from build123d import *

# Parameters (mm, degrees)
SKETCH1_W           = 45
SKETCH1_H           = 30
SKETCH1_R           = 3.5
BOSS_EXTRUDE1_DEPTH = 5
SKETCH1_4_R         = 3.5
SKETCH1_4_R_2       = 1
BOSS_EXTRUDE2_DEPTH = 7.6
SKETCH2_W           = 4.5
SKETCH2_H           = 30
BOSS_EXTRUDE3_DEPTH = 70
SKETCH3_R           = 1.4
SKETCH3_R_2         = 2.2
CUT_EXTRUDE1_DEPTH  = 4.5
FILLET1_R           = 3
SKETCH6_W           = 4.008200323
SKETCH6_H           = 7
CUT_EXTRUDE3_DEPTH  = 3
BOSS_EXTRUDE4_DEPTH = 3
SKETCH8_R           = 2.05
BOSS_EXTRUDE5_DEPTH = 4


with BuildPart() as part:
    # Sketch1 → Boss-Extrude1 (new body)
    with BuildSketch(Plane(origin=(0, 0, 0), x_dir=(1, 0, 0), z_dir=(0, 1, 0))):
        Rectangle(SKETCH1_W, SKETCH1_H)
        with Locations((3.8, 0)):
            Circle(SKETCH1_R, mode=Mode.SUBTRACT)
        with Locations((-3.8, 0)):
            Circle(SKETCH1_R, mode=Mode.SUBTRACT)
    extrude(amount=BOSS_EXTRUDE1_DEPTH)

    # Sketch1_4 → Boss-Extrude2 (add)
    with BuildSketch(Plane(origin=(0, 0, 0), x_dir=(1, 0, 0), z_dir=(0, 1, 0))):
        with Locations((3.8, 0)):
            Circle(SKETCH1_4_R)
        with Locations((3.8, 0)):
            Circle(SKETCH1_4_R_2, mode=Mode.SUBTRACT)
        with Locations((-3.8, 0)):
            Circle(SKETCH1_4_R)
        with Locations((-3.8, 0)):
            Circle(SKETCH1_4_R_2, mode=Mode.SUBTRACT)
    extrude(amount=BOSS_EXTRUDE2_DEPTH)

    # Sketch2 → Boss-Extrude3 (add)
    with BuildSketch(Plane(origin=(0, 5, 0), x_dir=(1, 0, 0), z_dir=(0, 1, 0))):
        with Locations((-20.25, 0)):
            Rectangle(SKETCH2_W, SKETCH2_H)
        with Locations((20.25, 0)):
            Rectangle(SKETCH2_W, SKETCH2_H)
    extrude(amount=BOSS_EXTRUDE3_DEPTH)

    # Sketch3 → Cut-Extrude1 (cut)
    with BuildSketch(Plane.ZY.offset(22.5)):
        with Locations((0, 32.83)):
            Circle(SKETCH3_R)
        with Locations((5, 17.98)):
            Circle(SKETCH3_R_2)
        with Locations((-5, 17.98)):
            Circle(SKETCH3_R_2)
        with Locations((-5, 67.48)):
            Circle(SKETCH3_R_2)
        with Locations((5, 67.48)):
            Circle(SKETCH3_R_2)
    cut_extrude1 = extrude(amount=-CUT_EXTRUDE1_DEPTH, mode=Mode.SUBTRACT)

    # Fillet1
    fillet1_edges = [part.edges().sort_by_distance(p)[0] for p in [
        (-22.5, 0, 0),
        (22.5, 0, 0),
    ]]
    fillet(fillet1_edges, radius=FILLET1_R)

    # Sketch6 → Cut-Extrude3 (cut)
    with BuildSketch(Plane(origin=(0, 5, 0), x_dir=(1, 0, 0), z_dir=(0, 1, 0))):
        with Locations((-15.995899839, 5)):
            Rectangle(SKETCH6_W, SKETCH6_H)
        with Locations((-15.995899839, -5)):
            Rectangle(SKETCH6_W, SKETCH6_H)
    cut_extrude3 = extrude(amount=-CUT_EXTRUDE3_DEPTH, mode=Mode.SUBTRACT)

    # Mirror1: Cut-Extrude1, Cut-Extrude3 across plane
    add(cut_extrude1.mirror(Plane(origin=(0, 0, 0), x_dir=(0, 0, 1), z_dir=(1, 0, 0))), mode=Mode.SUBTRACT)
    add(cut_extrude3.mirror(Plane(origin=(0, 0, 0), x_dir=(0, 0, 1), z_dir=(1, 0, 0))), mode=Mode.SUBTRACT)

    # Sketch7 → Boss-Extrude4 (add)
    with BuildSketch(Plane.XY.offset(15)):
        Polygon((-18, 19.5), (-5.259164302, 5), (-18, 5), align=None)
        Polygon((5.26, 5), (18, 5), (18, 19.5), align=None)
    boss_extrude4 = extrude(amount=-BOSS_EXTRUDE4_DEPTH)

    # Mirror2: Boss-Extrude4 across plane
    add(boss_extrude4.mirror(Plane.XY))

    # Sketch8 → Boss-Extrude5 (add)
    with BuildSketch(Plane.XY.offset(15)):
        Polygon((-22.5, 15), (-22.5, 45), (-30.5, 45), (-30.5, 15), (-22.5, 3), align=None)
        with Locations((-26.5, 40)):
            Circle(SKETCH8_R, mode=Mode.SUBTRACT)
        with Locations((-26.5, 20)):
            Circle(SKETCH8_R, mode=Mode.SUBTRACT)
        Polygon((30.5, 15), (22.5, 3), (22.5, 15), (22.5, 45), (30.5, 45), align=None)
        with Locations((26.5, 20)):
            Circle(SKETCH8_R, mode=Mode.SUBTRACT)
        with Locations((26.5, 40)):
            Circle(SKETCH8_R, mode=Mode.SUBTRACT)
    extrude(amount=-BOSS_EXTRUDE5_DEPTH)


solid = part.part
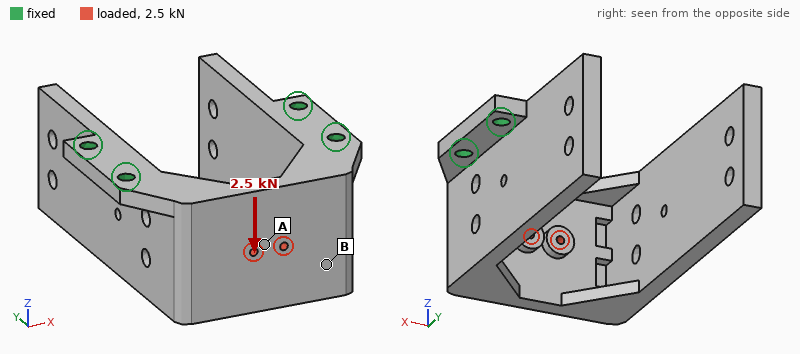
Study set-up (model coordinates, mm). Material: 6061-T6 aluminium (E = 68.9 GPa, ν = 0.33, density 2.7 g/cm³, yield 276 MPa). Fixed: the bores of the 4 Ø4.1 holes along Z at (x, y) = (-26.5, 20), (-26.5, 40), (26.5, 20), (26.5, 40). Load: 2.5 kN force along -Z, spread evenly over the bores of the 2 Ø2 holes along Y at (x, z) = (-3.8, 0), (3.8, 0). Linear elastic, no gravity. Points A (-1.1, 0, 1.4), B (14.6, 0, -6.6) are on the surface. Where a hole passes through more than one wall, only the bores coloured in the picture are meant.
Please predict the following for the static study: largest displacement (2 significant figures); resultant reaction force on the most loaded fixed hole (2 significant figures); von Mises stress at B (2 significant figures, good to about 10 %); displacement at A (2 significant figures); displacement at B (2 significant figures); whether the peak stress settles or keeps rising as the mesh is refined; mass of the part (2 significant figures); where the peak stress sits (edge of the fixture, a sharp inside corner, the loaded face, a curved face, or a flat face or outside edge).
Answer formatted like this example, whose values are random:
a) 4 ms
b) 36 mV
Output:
a) 82 µm
b) 2.1 kN
c) 28 MPa
d) 72 µm
e) 69 µm
f) keeps rising
g) 75 g
h) edge of the fixture
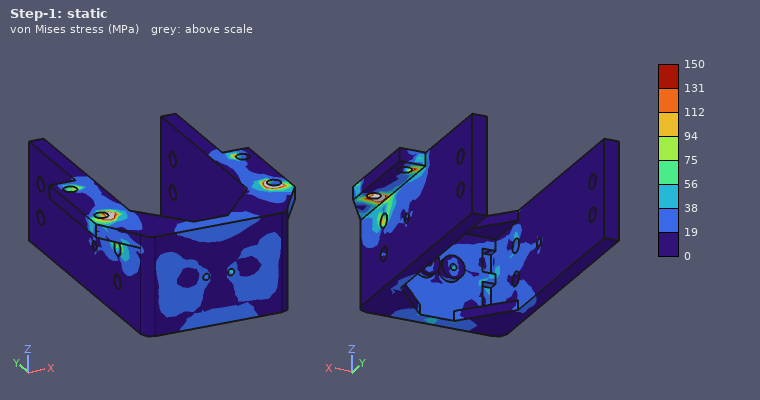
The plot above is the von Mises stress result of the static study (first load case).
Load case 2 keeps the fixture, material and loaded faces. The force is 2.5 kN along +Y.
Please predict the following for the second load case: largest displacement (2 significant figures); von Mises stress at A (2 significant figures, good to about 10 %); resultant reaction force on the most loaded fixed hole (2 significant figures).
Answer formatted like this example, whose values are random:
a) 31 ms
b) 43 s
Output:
a) 79 µm
b) 89 MPa
c) 1.1 kN
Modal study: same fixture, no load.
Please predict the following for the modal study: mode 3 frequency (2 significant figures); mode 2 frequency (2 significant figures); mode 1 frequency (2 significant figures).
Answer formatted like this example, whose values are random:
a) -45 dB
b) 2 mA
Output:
a) 4100 Hz
b) 2000 Hz
c) 2000 Hz
